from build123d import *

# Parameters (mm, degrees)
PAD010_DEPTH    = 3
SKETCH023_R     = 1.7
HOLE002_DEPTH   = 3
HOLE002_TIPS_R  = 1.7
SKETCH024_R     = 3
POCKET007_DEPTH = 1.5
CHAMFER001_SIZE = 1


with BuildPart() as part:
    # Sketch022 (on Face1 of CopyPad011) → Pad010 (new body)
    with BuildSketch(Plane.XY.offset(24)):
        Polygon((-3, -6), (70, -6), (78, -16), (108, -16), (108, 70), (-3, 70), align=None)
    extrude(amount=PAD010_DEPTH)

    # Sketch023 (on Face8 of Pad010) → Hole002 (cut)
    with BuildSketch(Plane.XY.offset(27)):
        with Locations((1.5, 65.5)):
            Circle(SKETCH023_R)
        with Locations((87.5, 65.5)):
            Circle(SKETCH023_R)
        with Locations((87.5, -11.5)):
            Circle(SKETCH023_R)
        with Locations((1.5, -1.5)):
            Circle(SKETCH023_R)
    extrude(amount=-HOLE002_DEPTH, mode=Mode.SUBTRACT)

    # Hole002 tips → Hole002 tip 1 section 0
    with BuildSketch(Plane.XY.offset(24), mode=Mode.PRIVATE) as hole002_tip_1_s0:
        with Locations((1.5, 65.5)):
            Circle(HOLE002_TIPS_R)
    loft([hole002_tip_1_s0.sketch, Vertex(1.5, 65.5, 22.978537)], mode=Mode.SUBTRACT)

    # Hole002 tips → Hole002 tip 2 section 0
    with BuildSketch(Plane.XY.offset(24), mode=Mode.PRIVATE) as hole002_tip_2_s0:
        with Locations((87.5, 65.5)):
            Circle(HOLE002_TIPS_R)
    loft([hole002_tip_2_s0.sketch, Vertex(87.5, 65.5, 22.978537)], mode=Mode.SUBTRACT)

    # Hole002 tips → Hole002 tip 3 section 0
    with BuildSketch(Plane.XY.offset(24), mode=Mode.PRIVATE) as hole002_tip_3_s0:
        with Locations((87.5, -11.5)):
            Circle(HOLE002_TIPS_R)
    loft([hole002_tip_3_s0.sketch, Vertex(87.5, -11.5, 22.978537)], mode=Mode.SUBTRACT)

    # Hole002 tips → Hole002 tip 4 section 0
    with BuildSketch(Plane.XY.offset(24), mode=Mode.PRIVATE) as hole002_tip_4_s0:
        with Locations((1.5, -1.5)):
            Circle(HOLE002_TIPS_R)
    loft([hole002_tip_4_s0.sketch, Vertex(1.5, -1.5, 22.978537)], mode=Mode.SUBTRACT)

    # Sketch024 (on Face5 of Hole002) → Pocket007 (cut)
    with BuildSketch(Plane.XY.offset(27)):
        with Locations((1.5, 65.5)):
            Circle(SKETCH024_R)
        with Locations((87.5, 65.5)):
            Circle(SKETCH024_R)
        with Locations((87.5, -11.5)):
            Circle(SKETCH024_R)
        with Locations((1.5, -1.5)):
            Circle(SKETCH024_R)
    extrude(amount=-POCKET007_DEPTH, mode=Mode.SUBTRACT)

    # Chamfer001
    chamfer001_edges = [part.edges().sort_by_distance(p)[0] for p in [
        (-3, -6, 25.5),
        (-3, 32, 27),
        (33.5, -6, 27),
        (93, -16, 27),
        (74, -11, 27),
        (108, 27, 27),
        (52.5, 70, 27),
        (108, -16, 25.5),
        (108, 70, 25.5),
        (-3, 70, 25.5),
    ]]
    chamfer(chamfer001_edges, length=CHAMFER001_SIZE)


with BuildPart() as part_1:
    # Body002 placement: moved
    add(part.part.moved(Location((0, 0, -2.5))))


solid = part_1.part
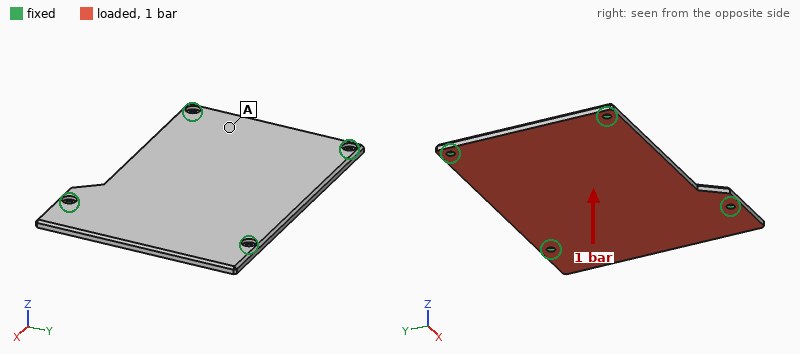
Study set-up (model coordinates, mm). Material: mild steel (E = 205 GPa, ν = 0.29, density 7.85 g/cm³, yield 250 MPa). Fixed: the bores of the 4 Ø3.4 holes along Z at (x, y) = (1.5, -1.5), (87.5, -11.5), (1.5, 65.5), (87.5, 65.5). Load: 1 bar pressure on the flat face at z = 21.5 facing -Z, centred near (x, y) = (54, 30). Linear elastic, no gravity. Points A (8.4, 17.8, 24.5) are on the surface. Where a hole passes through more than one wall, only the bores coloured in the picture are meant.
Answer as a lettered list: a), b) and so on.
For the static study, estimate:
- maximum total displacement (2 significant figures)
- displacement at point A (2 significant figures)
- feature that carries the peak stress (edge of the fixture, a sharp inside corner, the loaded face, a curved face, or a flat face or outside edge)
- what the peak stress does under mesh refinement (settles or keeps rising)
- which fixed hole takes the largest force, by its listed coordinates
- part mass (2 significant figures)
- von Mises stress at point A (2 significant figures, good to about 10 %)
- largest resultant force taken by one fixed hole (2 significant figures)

a) 84 µm
b) 32 µm
c) edge of the fixture
d) keeps rising
e) (87.5, 65.5)
f) 200 g
g) 19 MPa
h) 580 N
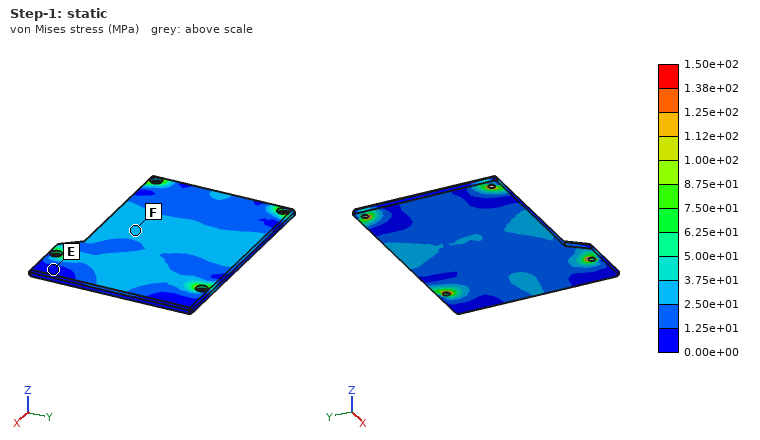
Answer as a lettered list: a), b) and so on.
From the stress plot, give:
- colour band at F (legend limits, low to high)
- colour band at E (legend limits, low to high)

a) 2.50e+01 to 3.75e+01 MPa
b) 0.00e+00 to 1.25e+01 MPa
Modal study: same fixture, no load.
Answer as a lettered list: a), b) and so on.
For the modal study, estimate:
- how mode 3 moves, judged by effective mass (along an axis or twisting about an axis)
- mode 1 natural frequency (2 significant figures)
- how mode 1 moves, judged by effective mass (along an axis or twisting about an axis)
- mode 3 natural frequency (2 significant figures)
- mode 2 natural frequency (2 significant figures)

a) twisting about X
b) 1300 Hz
c) along Z
d) 2300 Hz
e) 1900 Hz
